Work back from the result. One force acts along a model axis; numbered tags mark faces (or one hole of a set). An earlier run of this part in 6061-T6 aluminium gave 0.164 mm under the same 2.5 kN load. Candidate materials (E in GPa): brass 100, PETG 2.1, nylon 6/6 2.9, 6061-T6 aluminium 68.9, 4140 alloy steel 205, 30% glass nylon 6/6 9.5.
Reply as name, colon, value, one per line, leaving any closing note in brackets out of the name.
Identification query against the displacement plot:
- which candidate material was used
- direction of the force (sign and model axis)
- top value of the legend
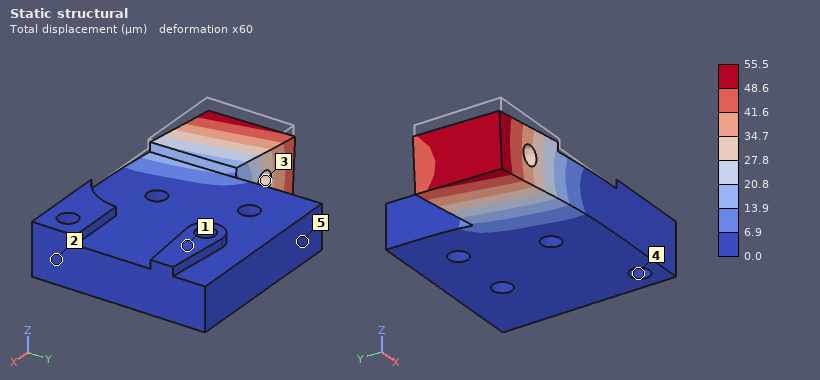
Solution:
which candidate material was used: 4140 alloy steel
direction of the force: -Z
top value of the legend: 55.5 µm
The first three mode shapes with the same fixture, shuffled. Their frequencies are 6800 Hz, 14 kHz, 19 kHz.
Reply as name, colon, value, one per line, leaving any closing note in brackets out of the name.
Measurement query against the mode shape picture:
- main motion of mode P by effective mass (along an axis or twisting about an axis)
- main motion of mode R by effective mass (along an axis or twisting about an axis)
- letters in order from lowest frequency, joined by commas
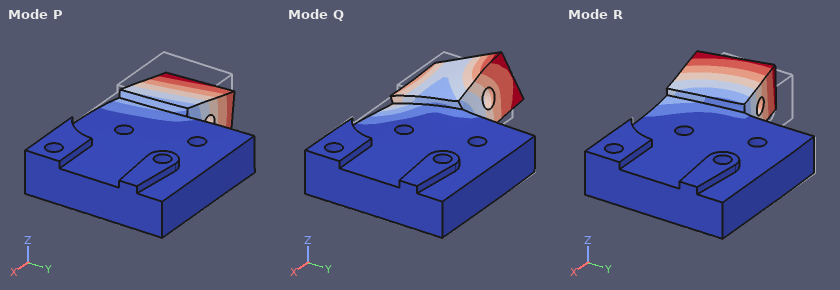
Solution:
main motion of mode P by effective mass: along Z
main motion of mode R by effective mass: along Y
letters in order from lowest frequency, joined by commas: P, R, Q
